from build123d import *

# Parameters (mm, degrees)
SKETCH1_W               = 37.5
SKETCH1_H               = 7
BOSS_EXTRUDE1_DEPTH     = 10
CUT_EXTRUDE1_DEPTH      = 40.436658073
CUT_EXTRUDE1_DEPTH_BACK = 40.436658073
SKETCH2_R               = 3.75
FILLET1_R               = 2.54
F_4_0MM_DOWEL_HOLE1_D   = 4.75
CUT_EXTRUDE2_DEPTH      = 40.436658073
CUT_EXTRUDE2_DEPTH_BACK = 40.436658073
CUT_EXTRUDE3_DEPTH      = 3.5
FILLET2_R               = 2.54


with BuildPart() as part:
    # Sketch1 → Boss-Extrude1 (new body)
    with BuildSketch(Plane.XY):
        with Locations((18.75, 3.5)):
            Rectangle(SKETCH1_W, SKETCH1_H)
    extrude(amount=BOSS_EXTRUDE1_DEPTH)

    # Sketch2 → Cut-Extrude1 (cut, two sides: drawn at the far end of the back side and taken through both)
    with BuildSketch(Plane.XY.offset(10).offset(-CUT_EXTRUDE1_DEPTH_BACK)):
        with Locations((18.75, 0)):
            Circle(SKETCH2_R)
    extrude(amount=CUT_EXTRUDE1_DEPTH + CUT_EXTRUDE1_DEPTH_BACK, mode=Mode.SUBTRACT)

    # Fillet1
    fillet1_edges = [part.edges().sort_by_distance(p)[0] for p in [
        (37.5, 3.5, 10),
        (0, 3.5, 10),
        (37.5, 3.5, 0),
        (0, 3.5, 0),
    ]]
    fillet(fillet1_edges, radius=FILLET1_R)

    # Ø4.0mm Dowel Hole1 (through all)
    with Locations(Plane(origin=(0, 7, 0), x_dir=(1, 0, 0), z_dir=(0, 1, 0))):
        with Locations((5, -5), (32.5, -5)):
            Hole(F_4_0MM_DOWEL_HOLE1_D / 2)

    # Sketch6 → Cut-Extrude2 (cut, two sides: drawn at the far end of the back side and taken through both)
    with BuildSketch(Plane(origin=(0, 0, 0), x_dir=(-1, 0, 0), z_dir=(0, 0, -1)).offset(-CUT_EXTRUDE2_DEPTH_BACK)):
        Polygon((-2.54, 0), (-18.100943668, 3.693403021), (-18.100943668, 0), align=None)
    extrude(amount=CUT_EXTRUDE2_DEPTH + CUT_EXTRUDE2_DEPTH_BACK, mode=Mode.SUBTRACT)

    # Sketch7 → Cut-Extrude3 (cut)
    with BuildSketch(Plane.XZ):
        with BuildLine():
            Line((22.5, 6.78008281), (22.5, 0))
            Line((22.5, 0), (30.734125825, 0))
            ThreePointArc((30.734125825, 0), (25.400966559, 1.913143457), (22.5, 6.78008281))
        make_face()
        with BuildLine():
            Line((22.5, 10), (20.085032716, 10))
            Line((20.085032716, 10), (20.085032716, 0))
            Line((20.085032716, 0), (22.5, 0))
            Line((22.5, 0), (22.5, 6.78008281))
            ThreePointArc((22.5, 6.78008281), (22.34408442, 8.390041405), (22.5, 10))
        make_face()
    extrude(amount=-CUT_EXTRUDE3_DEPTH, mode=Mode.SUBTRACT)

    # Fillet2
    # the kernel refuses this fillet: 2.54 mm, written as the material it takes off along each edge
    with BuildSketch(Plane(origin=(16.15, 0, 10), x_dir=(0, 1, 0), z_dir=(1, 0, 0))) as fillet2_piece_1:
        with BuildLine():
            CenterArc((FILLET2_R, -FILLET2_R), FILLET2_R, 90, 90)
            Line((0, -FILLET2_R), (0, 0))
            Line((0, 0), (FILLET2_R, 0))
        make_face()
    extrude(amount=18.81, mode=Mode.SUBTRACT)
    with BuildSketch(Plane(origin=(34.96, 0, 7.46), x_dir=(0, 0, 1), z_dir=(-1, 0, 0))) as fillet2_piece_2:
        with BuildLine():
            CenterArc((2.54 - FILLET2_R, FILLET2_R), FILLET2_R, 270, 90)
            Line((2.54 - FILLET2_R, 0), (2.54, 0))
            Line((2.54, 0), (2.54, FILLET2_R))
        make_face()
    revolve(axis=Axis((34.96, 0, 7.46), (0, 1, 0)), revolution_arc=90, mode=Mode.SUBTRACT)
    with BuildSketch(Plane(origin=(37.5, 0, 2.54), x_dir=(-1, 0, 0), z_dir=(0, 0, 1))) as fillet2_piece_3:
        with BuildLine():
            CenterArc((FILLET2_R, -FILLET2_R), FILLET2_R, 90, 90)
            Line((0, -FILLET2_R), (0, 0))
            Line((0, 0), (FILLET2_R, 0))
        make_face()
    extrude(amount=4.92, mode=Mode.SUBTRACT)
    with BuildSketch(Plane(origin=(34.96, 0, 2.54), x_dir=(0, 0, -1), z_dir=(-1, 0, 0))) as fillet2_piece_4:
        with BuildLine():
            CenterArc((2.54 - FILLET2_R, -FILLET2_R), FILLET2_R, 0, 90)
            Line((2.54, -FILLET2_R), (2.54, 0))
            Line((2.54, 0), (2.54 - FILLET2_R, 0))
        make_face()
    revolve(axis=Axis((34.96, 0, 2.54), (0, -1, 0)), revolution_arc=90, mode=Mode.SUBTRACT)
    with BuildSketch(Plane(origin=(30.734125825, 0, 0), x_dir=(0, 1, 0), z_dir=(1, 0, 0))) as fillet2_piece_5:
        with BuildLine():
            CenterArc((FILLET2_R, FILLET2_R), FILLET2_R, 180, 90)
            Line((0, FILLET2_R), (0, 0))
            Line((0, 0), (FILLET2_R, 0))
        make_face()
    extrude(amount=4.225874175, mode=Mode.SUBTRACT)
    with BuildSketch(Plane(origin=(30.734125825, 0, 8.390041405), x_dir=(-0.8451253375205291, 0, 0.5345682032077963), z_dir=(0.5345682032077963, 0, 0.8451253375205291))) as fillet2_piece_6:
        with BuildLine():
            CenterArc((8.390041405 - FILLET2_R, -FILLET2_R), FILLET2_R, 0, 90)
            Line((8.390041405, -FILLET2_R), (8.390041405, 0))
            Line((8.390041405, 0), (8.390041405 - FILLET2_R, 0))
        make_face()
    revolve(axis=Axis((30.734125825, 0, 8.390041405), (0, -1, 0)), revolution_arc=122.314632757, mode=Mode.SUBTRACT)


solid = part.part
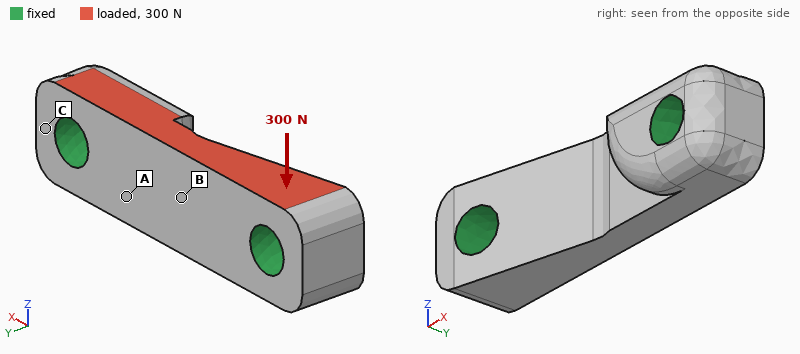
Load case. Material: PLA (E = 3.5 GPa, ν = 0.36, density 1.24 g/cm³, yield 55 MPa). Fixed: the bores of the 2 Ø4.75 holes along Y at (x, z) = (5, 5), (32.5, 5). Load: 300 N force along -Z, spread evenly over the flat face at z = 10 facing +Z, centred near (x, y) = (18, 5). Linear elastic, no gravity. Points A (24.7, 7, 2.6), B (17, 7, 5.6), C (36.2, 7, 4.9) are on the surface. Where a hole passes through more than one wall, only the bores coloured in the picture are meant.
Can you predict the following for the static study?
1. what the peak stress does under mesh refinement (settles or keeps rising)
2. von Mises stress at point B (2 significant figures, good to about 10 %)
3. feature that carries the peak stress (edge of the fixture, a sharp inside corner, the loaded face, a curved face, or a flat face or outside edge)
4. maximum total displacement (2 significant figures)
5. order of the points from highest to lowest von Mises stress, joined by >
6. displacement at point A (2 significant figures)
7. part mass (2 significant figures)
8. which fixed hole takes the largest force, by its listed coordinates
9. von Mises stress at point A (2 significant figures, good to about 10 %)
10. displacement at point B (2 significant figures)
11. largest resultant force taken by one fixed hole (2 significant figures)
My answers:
keeps rising
1.7 MPa
edge of the fixture
25 µm
A > B > C
15 µm
2.2 g
(5, 5)
3.0 MPa
22 µm
160 N
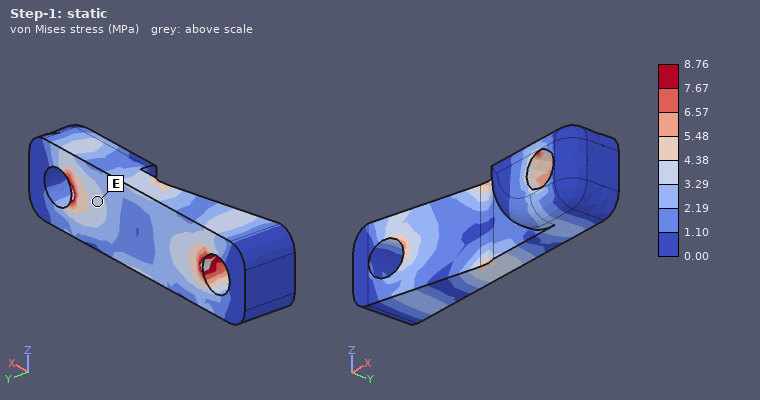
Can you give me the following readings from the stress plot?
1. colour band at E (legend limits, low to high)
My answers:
3.29 to 4.38 MPa
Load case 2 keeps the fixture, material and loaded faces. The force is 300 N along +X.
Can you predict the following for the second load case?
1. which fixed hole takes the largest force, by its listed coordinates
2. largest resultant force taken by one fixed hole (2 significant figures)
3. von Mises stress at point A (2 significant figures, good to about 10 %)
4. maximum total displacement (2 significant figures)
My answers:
(5, 5)
170 N
0.98 MPa
9.9 µm
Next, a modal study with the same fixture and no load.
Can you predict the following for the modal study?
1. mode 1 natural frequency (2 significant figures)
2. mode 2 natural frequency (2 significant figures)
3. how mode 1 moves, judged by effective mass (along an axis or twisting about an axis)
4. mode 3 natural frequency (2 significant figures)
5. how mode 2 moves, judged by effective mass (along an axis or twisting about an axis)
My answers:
14 kHz
15 kHz
along Y
21 kHz
along Z
